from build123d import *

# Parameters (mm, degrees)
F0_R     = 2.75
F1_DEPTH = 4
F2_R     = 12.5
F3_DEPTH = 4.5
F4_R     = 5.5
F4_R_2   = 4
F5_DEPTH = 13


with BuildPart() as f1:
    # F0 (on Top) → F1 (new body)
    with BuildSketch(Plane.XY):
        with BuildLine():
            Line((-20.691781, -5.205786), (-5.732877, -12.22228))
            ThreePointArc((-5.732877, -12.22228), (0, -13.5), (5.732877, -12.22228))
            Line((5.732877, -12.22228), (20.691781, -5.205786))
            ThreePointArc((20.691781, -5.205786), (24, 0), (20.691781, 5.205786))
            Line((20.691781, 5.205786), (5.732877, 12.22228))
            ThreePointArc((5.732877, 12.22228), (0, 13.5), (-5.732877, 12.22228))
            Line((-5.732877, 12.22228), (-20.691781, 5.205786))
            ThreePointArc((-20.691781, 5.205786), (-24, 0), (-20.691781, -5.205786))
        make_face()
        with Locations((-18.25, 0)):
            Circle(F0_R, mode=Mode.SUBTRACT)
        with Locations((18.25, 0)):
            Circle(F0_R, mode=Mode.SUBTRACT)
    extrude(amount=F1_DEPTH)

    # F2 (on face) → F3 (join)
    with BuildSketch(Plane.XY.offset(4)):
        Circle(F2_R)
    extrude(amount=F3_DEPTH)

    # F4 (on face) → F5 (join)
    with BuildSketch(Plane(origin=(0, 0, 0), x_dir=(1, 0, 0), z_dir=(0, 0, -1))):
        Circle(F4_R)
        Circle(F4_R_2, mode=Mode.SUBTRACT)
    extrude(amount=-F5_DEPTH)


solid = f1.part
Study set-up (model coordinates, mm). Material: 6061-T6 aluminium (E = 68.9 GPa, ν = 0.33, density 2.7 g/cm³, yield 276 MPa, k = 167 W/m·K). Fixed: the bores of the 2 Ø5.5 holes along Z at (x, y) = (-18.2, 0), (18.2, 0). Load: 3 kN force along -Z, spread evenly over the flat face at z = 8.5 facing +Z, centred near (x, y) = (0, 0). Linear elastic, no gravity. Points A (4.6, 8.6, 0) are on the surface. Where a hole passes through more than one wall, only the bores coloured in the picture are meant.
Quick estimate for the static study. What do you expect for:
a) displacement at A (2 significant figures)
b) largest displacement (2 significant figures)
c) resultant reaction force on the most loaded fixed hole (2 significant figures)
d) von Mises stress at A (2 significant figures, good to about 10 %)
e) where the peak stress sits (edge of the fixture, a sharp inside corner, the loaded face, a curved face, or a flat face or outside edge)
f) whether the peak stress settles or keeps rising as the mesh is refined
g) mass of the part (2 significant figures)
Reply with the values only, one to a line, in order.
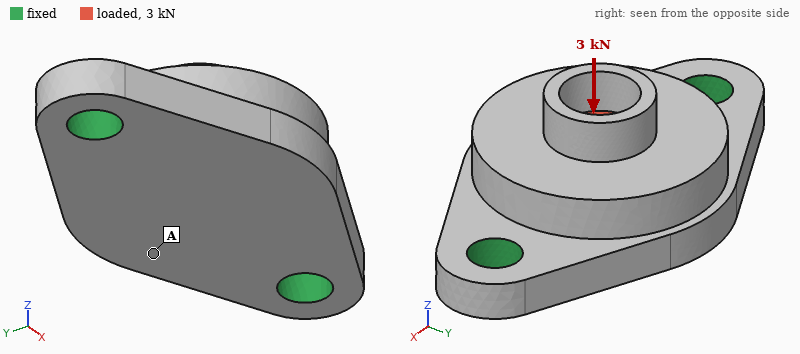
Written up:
25 µm
30 µm
1.8 kN
31 MPa
edge of the fixture
keeps rising
15 g
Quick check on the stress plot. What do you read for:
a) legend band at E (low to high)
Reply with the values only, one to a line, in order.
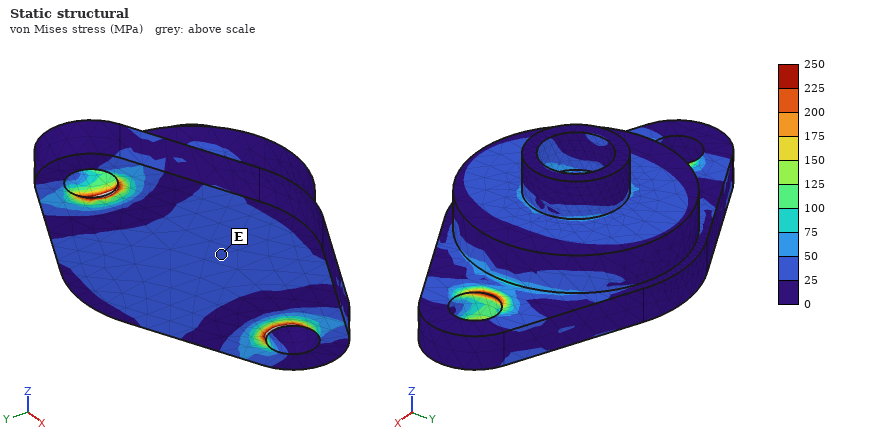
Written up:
25 to 50 MPa
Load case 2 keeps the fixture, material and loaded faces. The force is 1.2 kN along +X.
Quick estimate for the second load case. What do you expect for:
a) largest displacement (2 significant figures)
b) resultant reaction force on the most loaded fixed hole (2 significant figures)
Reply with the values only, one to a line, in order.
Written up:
4.8 µm
660 N
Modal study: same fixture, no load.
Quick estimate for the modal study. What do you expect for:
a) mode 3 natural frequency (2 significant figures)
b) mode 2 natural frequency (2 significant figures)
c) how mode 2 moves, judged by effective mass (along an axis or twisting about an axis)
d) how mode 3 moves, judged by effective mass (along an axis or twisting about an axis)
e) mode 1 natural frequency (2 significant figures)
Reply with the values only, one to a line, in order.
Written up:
26 kHz
16 kHz
along Z
along Y
11 kHz
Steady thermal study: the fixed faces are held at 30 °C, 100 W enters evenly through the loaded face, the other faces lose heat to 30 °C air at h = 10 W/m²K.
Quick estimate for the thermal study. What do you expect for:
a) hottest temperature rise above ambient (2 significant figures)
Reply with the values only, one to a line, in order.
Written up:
79 K
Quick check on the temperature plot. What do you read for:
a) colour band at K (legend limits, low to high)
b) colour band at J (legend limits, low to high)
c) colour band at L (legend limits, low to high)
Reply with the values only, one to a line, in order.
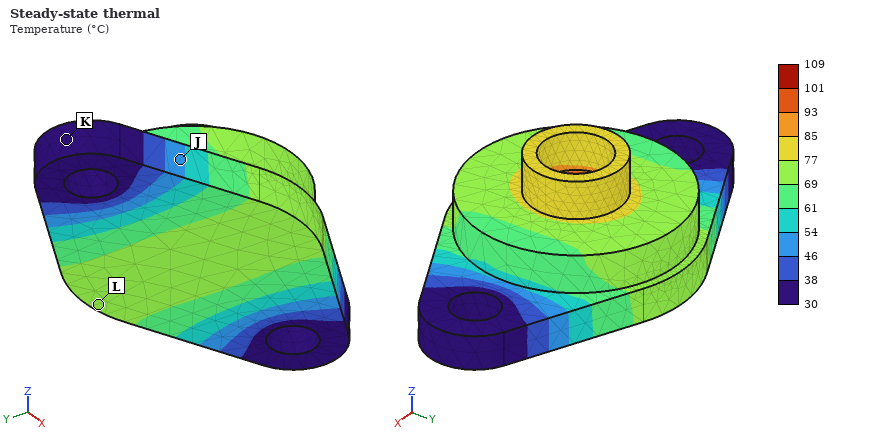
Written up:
30 to 38 °C
46 to 54 °C
69 to 77 °C
